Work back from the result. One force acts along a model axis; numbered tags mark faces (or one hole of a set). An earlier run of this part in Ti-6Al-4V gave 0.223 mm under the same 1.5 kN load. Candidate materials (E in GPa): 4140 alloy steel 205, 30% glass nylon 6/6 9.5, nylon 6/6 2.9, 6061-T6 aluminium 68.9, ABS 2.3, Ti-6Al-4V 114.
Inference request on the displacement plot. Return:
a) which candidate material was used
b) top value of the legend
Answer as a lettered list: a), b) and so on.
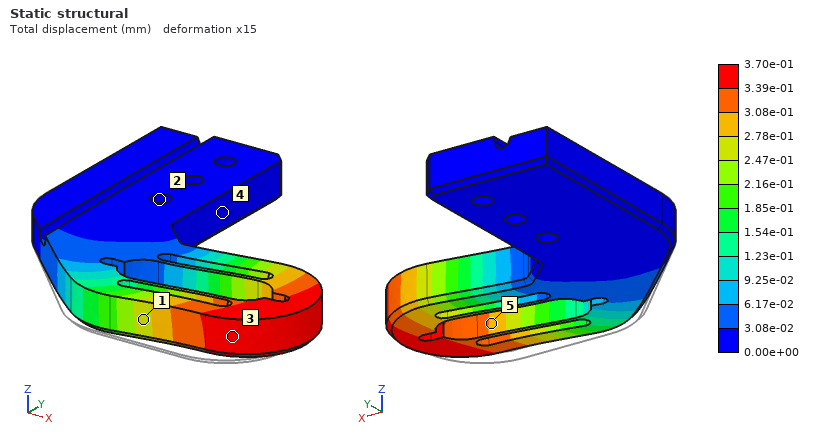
a) 6061-T6 aluminium
b) 3.70e-01 mm
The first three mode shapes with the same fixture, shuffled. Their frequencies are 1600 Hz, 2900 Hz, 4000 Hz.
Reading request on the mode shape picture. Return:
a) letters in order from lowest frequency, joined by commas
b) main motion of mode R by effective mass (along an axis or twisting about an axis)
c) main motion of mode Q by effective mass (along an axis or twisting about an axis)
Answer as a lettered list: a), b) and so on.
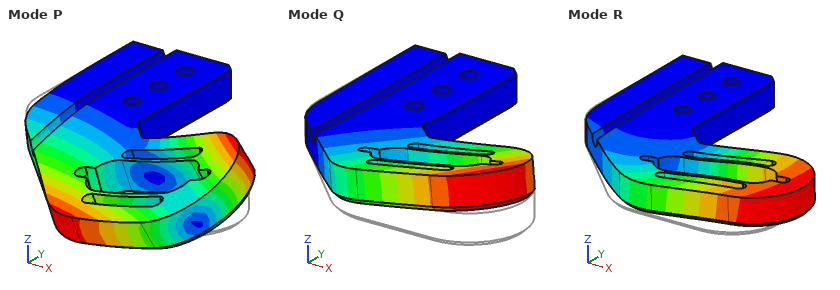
a) Q, R, P
b) along Y
c) along Z
